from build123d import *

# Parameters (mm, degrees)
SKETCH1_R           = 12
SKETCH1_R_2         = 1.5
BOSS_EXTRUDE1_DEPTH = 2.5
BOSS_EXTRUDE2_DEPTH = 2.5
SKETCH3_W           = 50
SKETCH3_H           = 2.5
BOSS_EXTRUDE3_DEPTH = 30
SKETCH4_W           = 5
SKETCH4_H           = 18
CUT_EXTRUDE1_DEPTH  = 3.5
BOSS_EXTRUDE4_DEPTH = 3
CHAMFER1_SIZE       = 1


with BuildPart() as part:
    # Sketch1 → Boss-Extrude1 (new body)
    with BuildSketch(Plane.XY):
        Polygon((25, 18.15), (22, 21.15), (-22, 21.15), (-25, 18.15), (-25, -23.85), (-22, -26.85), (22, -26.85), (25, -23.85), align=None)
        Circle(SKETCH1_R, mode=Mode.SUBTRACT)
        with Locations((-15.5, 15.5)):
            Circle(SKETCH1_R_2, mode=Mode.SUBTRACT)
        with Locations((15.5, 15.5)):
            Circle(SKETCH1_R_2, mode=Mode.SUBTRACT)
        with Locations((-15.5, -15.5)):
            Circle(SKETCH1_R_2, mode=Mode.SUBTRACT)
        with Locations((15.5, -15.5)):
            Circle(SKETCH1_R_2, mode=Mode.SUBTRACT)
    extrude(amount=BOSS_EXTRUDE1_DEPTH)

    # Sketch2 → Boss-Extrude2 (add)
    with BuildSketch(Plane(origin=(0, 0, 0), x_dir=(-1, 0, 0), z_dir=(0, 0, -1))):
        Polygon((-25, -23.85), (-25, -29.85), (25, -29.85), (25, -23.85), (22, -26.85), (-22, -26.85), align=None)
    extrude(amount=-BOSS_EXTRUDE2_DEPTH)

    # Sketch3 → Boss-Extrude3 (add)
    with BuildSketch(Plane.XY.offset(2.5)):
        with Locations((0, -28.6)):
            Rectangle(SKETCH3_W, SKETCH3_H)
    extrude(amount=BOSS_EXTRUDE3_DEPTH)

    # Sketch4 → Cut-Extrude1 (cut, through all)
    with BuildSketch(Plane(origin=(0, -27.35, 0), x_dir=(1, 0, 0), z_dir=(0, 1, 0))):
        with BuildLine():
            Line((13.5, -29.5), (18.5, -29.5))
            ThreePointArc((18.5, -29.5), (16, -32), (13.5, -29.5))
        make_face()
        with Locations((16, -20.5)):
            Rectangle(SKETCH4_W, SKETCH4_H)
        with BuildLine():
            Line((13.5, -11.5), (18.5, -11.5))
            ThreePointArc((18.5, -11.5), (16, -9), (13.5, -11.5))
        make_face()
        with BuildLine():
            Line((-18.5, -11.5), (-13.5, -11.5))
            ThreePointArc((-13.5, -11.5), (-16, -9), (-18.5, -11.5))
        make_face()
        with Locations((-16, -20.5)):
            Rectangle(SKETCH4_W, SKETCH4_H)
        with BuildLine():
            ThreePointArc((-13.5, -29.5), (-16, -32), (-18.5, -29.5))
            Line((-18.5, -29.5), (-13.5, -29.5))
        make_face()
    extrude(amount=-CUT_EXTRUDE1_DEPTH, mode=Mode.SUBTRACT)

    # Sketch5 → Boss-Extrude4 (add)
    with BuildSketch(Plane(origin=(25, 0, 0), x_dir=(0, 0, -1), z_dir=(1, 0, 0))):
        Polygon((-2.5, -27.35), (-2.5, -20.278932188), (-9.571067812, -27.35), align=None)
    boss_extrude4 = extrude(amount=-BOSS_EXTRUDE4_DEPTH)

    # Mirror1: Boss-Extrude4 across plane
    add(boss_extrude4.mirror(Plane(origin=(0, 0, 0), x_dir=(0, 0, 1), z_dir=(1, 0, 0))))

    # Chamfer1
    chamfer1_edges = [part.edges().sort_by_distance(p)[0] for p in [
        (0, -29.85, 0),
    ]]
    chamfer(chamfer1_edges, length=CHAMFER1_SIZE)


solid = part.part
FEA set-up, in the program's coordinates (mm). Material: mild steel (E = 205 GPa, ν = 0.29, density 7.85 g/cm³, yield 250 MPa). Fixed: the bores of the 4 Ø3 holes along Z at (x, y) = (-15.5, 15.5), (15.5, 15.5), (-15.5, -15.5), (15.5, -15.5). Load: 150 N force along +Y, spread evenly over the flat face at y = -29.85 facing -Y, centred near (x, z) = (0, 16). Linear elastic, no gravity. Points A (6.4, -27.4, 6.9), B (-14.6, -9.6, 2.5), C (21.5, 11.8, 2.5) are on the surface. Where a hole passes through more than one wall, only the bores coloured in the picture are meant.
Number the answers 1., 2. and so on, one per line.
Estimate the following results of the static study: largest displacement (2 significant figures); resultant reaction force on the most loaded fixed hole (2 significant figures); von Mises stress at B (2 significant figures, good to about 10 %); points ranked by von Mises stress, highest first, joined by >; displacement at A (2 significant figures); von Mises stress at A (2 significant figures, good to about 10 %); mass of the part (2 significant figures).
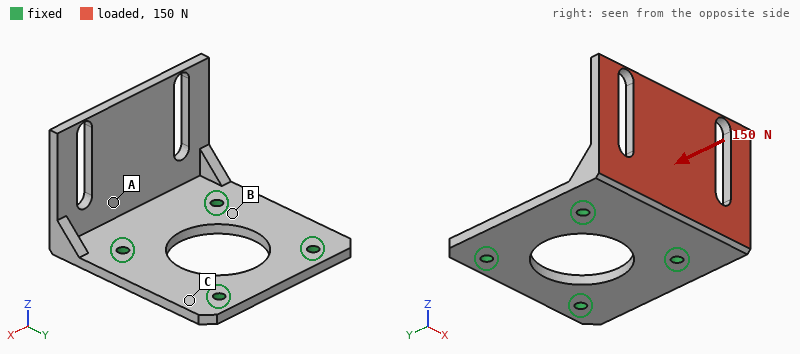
1. 95 µm
2. 69 N
3. 12 MPa
4. A > B > C
5. 17 µm
6. 23 MPa
7. 67 g
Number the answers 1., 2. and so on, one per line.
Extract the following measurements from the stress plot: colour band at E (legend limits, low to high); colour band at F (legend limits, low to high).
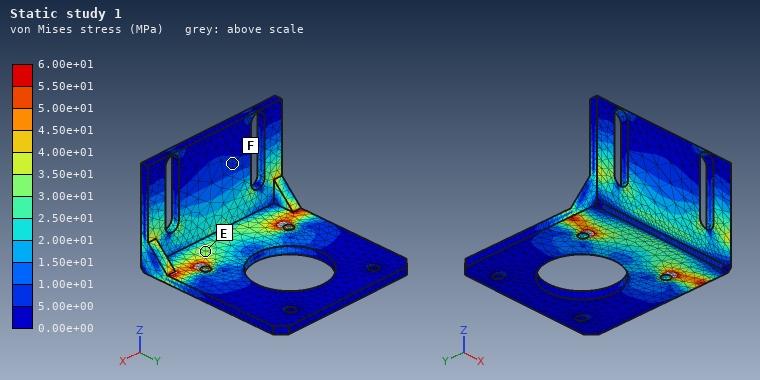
1. 3.00e+01 to 3.50e+01 MPa
2. 5.00e+00 to 1.00e+01 MPa
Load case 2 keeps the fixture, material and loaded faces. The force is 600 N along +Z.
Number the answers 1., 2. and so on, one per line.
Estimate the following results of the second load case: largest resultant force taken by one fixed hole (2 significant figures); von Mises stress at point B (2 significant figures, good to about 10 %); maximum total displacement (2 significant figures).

1. 320 N
2. 30 MPa
3. 0.17 mm
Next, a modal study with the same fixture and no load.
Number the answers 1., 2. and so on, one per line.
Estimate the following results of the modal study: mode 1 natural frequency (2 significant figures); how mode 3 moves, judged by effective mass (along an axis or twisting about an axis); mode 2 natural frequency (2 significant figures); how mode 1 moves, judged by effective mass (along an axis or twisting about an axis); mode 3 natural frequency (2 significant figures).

1. 1500 Hz
2. along Z
3. 2800 Hz
4. along Y
5. 4800 Hz
